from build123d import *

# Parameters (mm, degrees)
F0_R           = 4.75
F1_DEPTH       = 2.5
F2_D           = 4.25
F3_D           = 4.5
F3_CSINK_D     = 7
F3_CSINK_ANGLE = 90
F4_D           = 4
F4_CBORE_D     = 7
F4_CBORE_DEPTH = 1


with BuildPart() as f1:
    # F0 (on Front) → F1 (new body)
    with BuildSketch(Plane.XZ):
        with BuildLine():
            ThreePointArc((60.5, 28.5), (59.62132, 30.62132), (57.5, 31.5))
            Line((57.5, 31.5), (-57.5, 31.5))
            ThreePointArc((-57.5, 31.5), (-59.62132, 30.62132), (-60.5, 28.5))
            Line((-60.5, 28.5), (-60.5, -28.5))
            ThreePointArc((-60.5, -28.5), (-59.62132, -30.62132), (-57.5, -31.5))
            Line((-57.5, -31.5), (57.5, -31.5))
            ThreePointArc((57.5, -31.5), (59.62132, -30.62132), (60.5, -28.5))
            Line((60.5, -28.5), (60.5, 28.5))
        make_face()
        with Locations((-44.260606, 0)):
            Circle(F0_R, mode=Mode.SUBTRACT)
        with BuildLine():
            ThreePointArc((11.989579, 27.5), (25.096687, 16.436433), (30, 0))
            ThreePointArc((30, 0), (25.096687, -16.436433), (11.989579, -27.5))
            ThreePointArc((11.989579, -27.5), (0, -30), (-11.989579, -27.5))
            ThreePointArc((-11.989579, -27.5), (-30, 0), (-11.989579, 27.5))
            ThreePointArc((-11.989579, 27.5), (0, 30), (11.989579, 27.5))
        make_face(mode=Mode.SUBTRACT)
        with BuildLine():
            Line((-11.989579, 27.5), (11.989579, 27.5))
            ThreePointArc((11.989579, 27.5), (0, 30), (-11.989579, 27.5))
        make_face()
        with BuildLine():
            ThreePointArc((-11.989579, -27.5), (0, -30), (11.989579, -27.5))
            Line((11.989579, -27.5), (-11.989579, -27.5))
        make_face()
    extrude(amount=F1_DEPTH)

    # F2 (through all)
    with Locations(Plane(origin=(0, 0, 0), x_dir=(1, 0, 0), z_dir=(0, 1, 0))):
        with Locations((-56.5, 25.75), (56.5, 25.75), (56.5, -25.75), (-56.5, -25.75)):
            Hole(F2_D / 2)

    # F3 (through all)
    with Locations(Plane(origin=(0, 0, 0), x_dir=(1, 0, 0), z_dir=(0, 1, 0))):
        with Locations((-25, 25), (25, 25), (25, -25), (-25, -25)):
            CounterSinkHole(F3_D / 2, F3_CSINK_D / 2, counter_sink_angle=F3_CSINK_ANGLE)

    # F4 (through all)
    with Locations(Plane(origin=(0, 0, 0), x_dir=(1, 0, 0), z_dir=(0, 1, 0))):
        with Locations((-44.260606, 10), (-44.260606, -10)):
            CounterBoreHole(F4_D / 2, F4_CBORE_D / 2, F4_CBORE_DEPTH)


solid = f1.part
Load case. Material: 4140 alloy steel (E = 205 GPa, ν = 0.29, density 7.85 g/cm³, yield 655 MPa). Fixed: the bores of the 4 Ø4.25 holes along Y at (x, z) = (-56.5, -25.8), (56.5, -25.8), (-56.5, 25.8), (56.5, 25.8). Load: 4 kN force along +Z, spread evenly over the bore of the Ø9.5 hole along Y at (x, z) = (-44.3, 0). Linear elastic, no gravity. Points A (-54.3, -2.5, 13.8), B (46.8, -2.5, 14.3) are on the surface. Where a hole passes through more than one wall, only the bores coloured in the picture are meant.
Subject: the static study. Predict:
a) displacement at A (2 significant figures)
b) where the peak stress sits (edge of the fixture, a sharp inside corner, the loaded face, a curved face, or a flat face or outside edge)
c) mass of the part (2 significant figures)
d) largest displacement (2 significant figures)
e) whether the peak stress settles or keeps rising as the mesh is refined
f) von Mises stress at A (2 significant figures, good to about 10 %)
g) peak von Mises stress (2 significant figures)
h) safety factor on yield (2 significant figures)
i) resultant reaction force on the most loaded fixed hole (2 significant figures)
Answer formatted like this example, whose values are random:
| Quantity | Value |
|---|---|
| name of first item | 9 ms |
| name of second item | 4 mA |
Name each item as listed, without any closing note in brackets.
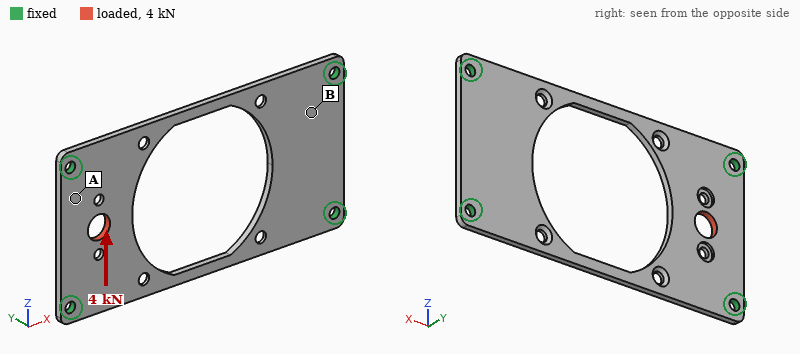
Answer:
| Quantity | Value |
|---|---|
| displacement at A | 3.8 µm |
| where the peak stress sits | a curved face |
| mass of the part | 90 g |
| largest displacement | 13 µm |
| whether the peak stress settles or keeps rising as the mesh is refined | settles |
| von Mises stress at A | 55 MPa |
| peak von Mises stress | 260 MPa |
| safety factor on yield | 2.6 |
| resultant reaction force on the most loaded fixed hole | 2.1 kN |
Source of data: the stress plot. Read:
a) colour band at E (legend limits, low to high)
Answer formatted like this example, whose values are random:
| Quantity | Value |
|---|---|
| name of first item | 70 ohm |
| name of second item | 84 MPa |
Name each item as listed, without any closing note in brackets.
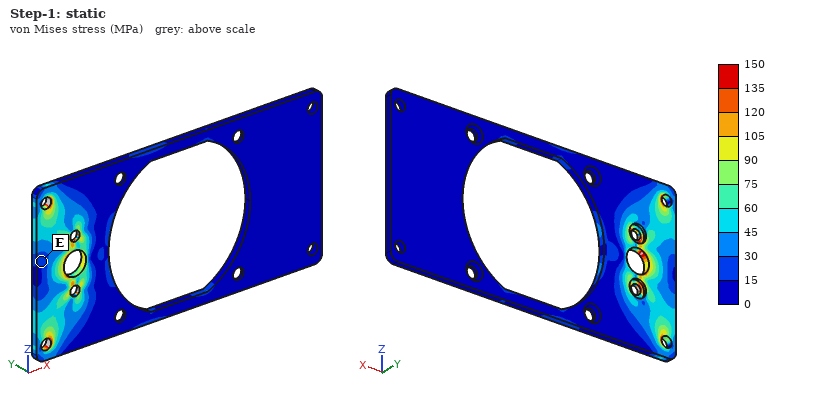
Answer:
| Quantity | Value |
|---|---|
| colour band at E | 15 to 30 MPa |
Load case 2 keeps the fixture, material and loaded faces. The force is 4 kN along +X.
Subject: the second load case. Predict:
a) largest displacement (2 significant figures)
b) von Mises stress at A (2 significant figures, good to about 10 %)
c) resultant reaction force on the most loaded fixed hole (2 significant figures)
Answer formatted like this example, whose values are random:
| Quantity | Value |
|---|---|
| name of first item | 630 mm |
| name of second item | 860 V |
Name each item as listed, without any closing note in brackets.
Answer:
| Quantity | Value |
|---|---|
| largest displacement | 17 µm |
| von Mises stress at A | 56 MPa |
| resultant reaction force on the most loaded fixed hole | 2.3 kN |
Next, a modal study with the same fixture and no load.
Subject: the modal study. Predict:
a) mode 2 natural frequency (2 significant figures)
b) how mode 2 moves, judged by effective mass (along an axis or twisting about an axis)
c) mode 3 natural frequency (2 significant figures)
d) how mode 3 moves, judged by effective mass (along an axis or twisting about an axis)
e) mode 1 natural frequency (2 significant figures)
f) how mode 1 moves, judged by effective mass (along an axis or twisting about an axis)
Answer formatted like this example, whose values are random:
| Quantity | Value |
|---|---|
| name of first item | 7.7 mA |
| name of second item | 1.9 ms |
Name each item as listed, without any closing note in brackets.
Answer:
| Quantity | Value |
|---|---|
| mode 2 natural frequency | 1800 Hz |
| how mode 2 moves, judged by effective mass | twisting about X |
| mode 3 natural frequency | 2200 Hz |
| how mode 3 moves, judged by effective mass | twisting about Z |
| mode 1 natural frequency | 1300 Hz |
| how mode 1 moves, judged by effective mass | along Y |
